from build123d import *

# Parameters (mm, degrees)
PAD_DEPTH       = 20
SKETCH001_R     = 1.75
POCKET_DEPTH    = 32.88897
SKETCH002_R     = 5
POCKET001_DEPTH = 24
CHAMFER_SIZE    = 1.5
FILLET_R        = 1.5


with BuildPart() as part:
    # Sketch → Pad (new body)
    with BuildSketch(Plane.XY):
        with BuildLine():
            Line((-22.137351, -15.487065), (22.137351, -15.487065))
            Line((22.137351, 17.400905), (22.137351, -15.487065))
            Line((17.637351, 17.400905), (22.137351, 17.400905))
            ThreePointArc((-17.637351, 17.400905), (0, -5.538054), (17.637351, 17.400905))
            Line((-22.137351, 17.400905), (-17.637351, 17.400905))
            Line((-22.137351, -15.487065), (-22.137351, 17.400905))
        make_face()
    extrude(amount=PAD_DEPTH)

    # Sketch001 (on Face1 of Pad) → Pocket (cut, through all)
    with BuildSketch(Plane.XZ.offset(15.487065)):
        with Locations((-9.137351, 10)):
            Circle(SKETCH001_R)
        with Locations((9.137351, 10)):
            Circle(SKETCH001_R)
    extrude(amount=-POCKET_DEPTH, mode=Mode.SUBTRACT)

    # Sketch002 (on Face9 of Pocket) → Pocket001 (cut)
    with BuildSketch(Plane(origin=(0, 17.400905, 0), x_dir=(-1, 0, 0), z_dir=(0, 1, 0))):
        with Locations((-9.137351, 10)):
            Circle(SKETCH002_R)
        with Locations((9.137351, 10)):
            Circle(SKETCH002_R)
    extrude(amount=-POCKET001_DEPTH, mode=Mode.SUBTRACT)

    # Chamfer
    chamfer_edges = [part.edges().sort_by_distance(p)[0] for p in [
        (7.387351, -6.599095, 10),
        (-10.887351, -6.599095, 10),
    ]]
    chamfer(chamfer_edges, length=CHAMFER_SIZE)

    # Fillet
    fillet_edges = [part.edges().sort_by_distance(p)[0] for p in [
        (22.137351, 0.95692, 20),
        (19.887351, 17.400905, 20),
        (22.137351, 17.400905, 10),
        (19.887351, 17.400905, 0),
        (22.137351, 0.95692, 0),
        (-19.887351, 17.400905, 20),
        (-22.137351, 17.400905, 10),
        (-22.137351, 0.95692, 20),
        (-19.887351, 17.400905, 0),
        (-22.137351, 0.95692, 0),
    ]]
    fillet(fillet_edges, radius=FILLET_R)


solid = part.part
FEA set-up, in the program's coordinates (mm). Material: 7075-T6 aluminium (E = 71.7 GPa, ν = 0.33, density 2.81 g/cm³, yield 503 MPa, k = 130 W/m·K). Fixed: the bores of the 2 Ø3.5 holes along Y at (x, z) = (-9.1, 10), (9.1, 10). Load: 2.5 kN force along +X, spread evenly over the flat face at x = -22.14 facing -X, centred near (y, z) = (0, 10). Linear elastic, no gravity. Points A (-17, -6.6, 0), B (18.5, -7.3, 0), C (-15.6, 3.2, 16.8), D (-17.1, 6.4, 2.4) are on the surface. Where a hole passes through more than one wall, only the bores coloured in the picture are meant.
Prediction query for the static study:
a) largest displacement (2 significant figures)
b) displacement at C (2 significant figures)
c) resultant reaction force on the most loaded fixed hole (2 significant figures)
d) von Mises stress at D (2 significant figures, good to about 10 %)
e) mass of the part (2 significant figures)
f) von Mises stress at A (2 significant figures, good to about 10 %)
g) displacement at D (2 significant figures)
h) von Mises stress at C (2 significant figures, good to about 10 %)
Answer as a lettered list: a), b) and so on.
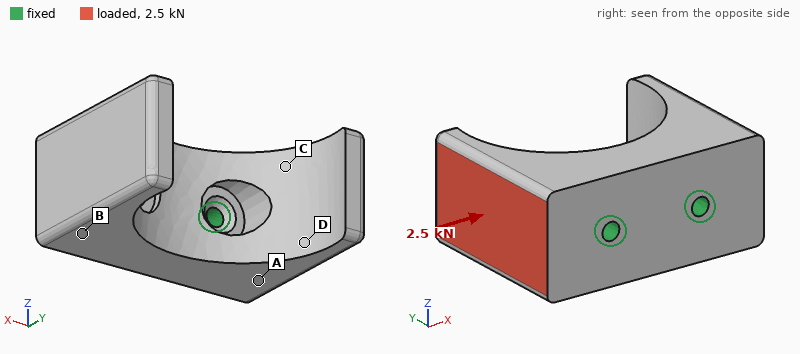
a) 0.11 mm
b) 0.035 mm
c) 1.7 kN
d) 54 MPa
e) 40 g
f) 24 MPa
g) 0.048 mm
h) 63 MPa
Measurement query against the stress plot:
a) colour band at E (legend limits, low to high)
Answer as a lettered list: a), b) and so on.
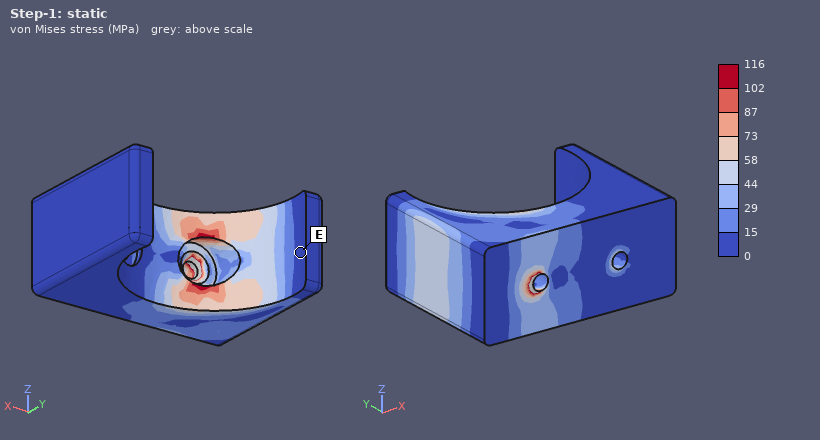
a) 0 to 15 MPa
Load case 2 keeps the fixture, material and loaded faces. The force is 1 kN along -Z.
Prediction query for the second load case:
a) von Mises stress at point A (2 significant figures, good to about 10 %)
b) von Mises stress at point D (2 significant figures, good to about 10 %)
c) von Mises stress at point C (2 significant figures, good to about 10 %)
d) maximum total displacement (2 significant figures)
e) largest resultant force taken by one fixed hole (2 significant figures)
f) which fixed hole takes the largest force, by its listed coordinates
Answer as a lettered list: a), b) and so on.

a) 8.1 MPa
b) 8.3 MPa
c) 12 MPa
d) 36 µm
e) 1.5 kN
f) (-9.1, 10)
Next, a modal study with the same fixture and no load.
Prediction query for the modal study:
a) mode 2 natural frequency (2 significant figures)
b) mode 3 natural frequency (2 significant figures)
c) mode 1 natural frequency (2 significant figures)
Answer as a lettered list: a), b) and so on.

a) 9400 Hz
b) 9400 Hz
c) 9300 Hz
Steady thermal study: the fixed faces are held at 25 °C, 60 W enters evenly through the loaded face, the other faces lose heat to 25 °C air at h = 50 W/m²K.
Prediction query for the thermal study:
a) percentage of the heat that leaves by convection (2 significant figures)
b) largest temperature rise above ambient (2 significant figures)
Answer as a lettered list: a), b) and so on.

a) 4.3 %
b) 50 K
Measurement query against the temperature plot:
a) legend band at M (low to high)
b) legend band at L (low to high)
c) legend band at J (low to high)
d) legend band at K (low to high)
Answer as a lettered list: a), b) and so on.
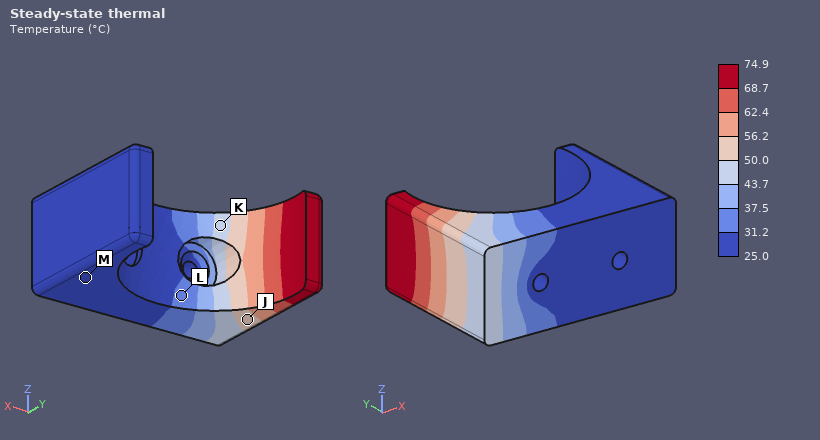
a) 25.0 to 31.2 °C
b) 31.2 to 37.5 °C
c) 50.0 to 56.2 °C
d) 43.7 to 50.0 °C
